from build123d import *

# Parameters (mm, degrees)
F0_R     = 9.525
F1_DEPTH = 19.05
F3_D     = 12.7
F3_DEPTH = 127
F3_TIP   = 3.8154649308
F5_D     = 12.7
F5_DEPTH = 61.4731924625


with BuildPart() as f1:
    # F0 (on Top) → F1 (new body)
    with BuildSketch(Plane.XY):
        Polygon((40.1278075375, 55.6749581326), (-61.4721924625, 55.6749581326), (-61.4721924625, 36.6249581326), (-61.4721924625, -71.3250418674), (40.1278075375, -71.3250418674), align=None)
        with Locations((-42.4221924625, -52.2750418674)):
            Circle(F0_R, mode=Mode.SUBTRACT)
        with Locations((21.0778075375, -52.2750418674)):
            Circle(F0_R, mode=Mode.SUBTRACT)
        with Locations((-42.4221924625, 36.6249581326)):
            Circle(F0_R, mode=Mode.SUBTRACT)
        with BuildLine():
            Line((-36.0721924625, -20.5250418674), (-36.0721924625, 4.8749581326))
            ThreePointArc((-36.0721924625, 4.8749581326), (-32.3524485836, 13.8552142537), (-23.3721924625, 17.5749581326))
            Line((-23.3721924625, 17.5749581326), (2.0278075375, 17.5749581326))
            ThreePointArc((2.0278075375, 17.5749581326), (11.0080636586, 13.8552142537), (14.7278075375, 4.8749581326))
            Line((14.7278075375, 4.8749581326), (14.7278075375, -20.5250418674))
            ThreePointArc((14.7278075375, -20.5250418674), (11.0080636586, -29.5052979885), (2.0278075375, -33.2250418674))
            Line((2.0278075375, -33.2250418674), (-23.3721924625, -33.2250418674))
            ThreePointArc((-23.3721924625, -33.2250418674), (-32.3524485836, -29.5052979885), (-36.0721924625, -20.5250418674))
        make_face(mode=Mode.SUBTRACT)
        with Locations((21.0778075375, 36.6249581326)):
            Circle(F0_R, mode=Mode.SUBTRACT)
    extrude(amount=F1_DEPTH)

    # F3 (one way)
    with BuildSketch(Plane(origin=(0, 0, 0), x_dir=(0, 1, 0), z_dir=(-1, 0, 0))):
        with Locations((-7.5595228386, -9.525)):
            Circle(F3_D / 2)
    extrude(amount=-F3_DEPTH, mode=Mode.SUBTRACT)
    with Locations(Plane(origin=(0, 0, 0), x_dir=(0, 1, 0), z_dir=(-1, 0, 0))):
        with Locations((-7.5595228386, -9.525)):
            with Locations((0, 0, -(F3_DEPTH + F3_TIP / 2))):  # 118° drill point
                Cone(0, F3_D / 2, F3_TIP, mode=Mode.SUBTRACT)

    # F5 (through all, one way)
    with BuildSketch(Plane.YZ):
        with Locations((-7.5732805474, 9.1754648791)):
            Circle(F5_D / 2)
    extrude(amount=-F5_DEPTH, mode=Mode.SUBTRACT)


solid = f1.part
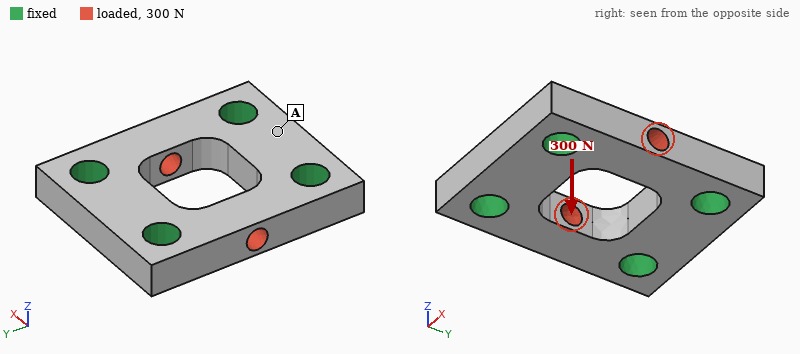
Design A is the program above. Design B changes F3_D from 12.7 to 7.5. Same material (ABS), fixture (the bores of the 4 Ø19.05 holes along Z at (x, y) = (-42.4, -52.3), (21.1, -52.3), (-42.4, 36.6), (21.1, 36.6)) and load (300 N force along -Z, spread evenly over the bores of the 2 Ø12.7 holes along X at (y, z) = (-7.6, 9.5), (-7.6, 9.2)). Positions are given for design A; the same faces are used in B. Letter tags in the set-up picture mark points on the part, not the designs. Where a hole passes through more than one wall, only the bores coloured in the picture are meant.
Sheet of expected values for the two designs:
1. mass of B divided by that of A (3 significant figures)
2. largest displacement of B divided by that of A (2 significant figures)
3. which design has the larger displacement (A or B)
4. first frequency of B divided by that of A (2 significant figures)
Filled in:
1.01
1.3
B
0.95
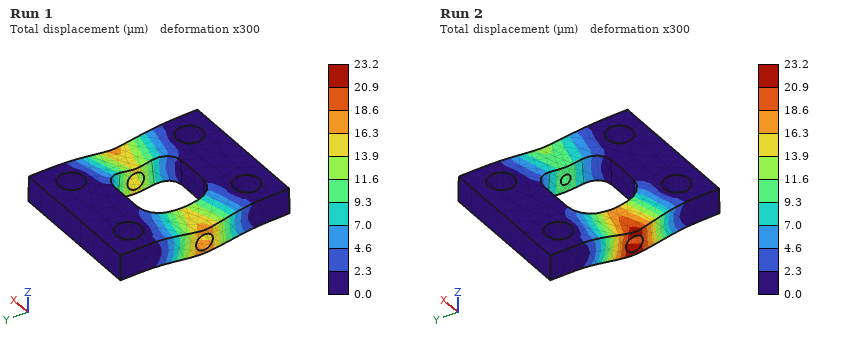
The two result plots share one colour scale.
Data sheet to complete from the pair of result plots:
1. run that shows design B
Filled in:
Run 2
